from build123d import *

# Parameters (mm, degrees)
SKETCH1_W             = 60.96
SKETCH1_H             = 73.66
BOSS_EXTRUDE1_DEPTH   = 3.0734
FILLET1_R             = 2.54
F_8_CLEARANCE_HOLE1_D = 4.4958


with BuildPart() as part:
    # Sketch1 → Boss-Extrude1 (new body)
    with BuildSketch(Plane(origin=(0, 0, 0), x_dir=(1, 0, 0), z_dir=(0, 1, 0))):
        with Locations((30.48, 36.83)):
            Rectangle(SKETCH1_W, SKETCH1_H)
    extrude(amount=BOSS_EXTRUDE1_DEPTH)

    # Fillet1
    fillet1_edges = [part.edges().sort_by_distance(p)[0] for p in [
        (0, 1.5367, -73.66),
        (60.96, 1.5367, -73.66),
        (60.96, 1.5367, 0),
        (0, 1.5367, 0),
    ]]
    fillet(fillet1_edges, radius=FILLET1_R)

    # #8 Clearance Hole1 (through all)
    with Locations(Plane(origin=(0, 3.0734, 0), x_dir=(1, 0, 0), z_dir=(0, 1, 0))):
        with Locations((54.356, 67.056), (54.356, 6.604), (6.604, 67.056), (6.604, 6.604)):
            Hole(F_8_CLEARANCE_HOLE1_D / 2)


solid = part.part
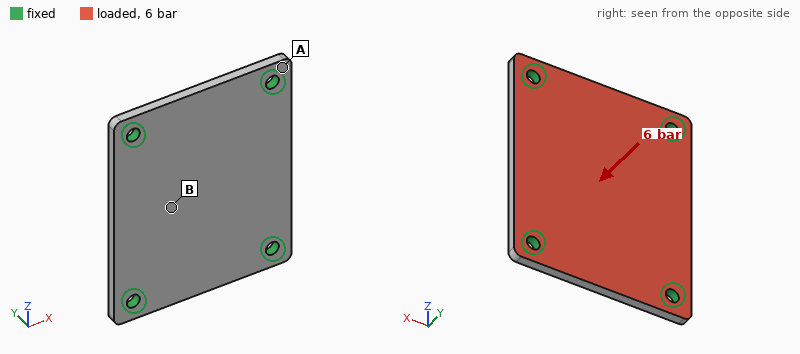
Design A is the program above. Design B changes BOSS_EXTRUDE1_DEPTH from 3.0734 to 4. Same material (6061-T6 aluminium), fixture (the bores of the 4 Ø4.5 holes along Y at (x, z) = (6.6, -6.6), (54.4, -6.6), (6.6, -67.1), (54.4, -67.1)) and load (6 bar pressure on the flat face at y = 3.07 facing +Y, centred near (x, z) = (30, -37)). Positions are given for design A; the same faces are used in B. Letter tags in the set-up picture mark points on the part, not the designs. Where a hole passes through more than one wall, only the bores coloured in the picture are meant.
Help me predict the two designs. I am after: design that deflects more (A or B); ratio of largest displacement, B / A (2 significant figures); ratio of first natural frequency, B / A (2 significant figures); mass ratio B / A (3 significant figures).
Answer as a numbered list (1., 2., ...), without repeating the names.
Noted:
1. A
2. 0.48
3. 1.3
4. 1.30
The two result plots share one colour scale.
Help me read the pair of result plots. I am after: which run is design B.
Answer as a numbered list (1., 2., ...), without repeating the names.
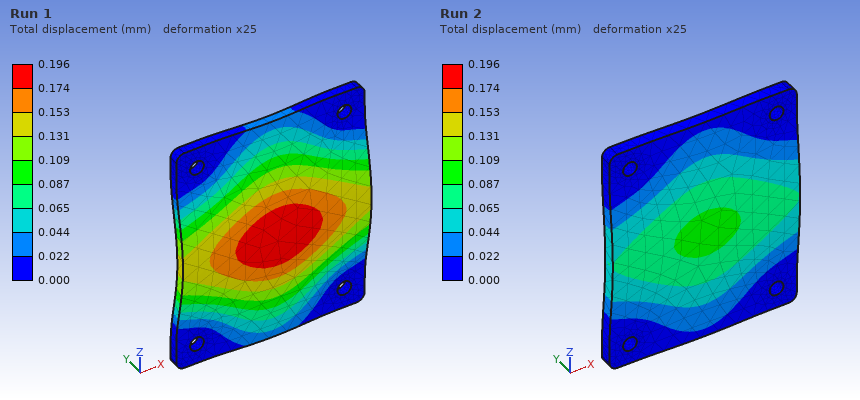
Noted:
1. Run 2
